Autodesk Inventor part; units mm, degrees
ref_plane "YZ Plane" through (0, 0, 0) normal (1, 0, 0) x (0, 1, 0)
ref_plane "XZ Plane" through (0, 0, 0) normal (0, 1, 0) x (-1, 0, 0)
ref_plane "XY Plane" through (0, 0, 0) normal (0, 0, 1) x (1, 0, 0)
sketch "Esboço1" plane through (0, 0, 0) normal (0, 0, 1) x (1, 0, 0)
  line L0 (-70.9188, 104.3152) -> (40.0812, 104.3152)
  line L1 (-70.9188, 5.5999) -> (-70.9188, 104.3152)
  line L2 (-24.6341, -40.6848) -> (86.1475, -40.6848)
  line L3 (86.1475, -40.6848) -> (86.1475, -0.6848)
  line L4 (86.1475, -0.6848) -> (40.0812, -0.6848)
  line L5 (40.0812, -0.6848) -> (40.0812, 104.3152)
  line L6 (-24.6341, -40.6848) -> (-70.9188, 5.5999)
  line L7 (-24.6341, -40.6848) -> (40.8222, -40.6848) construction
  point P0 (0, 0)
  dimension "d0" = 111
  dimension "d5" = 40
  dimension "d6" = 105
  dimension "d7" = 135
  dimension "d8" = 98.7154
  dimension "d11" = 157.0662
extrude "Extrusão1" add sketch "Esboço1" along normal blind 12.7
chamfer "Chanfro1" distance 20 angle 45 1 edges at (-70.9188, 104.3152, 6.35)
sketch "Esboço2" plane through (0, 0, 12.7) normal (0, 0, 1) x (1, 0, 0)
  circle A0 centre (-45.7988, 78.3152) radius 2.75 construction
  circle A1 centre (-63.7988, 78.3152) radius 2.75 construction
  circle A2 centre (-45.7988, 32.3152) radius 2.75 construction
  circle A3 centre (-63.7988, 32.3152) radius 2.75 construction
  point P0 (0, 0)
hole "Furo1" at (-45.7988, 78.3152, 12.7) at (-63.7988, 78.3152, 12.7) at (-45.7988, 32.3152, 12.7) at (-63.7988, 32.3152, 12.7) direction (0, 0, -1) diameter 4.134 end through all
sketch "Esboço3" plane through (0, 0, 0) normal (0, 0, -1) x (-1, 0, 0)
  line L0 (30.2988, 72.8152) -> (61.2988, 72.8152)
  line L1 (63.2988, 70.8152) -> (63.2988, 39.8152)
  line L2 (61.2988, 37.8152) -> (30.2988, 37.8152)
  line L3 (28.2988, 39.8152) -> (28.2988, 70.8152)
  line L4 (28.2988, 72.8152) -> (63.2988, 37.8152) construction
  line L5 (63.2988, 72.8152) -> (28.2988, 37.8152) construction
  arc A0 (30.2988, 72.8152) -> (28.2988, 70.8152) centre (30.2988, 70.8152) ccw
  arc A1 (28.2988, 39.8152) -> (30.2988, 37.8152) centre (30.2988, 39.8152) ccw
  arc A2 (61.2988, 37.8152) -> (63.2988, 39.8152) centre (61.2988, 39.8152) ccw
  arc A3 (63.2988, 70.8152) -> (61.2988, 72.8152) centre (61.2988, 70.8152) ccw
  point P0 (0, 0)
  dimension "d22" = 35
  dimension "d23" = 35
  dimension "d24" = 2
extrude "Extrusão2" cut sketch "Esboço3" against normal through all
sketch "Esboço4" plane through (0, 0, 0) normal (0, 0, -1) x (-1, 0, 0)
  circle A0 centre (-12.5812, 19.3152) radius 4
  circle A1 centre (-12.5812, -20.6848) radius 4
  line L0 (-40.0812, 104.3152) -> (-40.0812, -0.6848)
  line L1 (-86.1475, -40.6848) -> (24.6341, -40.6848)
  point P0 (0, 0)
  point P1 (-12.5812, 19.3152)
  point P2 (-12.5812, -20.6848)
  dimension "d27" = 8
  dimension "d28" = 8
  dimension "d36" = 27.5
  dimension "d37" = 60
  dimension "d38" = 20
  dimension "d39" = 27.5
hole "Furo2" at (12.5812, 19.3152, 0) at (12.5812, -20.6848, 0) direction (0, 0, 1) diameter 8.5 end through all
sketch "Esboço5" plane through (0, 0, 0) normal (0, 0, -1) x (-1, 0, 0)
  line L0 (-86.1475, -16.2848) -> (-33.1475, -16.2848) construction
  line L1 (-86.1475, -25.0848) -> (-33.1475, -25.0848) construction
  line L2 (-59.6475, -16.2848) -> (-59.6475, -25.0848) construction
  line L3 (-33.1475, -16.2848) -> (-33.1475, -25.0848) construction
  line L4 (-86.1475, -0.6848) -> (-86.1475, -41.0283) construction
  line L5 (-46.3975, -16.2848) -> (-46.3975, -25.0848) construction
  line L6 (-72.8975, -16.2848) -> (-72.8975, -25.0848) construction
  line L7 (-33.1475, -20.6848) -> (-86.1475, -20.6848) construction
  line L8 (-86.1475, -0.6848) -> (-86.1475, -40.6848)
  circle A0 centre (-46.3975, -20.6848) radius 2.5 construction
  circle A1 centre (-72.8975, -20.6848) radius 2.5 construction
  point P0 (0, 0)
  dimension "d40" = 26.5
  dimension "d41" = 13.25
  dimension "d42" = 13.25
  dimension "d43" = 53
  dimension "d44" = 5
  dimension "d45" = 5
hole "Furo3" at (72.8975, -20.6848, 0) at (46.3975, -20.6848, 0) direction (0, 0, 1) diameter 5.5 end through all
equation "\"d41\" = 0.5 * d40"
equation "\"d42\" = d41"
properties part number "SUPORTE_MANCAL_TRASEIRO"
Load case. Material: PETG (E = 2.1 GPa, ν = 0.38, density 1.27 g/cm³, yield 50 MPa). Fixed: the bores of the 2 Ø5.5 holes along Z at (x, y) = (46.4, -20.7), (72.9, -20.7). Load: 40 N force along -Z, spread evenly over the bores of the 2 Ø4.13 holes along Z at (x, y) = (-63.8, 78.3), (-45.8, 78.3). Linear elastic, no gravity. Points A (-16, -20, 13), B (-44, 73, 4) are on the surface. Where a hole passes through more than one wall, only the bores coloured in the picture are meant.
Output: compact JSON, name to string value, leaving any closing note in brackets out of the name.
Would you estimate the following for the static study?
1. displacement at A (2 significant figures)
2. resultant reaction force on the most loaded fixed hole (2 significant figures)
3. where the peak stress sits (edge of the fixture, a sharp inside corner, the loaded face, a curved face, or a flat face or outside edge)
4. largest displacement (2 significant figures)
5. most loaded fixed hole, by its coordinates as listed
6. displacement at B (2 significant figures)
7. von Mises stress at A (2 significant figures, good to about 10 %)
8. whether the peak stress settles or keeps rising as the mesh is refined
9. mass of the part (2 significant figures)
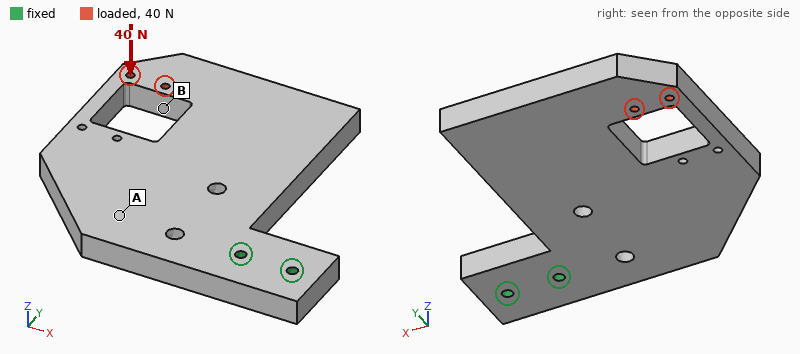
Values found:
{"displacement at A": "0.38 mm", "resultant reaction force on the most loaded fixed hole": "110 N", "where the peak stress sits": "edge of the fixture", "largest displacement": "2.4 mm", "most loaded fixed hole, by its coordinates as listed": "(46.4, -20.7)", "displacement at B": "1.9 mm", "von Mises stress at A": "1.3 MPa", "whether the peak stress settles or keeps rising as the mesh is refined": "keeps rising", "mass of the part": "250 g"}
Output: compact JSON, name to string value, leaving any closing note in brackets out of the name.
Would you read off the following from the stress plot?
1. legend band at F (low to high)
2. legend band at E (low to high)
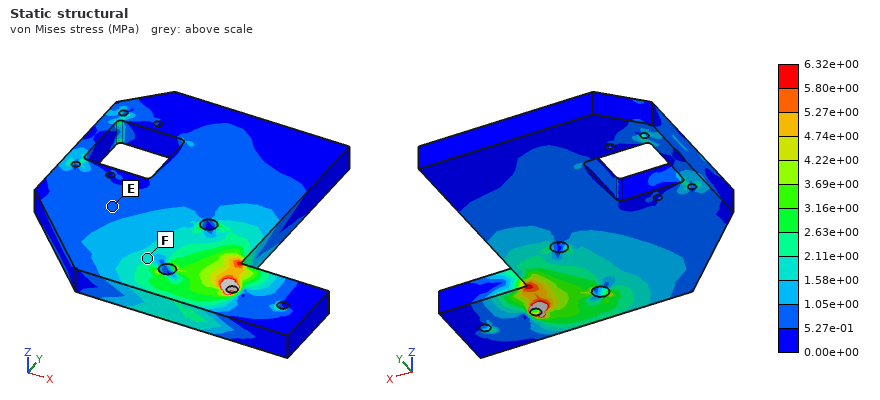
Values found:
{"legend band at F": "1.58e+00 to 2.11e+00 MPa", "legend band at E": "5.27e-01 to 1.05e+00 MPa"}
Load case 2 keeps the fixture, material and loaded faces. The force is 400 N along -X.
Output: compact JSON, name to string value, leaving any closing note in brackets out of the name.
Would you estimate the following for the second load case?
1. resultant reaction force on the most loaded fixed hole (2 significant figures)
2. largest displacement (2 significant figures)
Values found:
{"resultant reaction force on the most loaded fixed hole": "1.2 kN", "largest displacement": "2.3 mm"}
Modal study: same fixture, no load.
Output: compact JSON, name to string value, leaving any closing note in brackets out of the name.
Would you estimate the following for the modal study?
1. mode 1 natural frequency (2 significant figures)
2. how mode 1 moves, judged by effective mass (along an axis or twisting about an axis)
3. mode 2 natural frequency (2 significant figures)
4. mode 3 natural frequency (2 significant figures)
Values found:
{"mode 1 natural frequency": "87 Hz", "how mode 1 moves, judged by effective mass": "along Z", "mode 2 natural frequency": "190 Hz", "mode 3 natural frequency": "200 Hz"}
